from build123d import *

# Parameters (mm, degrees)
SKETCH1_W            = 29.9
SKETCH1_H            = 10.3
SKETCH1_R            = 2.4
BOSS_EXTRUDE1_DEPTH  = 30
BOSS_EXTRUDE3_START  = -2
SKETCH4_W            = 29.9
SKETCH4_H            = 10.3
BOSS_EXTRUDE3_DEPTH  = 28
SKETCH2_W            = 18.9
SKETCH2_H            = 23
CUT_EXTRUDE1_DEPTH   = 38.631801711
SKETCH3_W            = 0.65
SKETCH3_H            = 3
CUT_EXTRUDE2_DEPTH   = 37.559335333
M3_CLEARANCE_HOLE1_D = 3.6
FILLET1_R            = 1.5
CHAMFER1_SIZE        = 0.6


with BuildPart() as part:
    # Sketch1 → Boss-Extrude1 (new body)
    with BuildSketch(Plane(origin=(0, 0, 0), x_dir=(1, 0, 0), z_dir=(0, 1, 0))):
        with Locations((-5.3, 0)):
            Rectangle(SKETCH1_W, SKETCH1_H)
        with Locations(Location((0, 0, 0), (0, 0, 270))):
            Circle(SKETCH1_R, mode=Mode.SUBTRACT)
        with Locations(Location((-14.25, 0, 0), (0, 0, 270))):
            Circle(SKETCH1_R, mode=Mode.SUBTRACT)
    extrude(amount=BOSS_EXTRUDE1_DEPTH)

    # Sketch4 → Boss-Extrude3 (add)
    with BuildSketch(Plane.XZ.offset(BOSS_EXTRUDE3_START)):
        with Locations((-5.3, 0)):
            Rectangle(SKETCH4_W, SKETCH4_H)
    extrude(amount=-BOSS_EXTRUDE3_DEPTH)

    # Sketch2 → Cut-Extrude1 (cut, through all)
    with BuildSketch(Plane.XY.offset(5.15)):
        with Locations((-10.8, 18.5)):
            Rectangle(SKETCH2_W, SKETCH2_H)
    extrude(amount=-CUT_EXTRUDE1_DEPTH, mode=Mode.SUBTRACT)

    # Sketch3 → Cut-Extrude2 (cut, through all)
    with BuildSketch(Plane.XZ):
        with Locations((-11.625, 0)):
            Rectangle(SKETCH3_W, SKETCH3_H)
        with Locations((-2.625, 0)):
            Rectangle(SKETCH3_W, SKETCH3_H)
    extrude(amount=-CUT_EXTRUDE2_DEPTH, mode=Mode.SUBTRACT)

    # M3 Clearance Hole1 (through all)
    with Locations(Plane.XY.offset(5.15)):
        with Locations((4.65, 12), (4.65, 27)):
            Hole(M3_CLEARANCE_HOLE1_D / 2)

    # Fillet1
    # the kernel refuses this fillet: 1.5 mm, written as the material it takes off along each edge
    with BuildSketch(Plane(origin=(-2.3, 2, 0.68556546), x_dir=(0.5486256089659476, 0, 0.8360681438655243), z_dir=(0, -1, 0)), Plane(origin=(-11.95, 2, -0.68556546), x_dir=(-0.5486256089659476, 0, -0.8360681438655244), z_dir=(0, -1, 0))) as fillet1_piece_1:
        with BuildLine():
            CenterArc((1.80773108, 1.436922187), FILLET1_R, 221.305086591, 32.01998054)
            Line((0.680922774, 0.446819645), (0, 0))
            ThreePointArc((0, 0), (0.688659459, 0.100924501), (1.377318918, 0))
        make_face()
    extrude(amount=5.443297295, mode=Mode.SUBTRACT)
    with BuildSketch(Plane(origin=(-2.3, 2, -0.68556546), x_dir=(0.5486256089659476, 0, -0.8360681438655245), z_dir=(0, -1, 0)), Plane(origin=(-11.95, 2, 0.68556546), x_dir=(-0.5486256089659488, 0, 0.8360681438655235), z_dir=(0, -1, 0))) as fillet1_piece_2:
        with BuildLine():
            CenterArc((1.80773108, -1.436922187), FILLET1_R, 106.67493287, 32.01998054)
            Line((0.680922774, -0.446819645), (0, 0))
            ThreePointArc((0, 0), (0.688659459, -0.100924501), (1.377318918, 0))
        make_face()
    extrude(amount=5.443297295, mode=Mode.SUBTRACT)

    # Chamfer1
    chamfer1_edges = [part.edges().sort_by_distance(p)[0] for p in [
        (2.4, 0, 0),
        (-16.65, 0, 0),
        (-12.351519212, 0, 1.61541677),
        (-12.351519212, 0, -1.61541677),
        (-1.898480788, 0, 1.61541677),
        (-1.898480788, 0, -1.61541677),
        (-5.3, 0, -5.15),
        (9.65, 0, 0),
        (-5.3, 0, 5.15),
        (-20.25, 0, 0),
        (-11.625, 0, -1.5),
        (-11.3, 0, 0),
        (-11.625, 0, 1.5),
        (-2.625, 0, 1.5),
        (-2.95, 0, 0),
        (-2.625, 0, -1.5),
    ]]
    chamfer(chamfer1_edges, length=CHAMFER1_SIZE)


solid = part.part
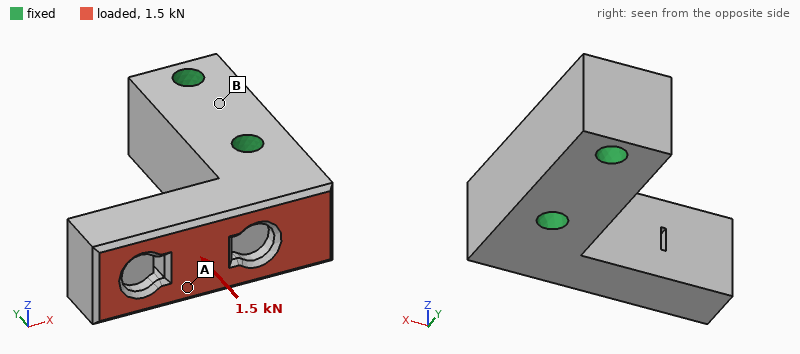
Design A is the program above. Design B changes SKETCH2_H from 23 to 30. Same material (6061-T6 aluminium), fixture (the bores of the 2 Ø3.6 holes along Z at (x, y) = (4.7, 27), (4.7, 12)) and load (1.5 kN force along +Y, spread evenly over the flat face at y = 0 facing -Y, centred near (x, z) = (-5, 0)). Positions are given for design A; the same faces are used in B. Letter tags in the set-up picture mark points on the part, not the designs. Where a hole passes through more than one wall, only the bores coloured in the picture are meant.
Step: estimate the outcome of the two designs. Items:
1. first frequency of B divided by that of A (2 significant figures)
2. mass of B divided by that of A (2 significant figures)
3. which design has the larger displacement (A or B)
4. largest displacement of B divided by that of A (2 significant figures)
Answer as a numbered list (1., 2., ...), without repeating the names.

1. 0.68
2. 0.85
3. B
4. 4.7
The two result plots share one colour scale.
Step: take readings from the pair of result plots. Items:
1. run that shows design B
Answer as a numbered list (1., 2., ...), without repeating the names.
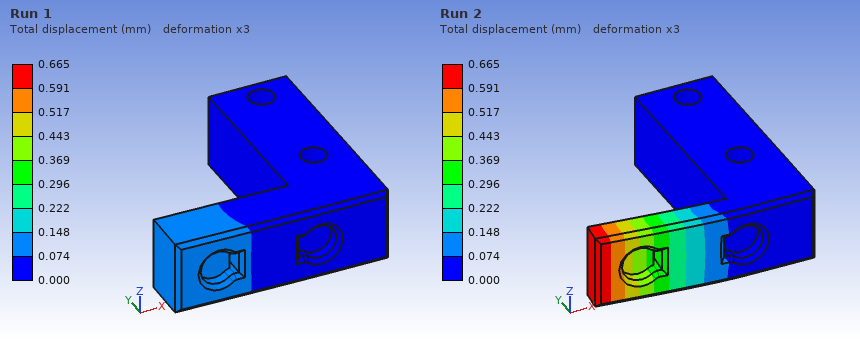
1. Run 2
